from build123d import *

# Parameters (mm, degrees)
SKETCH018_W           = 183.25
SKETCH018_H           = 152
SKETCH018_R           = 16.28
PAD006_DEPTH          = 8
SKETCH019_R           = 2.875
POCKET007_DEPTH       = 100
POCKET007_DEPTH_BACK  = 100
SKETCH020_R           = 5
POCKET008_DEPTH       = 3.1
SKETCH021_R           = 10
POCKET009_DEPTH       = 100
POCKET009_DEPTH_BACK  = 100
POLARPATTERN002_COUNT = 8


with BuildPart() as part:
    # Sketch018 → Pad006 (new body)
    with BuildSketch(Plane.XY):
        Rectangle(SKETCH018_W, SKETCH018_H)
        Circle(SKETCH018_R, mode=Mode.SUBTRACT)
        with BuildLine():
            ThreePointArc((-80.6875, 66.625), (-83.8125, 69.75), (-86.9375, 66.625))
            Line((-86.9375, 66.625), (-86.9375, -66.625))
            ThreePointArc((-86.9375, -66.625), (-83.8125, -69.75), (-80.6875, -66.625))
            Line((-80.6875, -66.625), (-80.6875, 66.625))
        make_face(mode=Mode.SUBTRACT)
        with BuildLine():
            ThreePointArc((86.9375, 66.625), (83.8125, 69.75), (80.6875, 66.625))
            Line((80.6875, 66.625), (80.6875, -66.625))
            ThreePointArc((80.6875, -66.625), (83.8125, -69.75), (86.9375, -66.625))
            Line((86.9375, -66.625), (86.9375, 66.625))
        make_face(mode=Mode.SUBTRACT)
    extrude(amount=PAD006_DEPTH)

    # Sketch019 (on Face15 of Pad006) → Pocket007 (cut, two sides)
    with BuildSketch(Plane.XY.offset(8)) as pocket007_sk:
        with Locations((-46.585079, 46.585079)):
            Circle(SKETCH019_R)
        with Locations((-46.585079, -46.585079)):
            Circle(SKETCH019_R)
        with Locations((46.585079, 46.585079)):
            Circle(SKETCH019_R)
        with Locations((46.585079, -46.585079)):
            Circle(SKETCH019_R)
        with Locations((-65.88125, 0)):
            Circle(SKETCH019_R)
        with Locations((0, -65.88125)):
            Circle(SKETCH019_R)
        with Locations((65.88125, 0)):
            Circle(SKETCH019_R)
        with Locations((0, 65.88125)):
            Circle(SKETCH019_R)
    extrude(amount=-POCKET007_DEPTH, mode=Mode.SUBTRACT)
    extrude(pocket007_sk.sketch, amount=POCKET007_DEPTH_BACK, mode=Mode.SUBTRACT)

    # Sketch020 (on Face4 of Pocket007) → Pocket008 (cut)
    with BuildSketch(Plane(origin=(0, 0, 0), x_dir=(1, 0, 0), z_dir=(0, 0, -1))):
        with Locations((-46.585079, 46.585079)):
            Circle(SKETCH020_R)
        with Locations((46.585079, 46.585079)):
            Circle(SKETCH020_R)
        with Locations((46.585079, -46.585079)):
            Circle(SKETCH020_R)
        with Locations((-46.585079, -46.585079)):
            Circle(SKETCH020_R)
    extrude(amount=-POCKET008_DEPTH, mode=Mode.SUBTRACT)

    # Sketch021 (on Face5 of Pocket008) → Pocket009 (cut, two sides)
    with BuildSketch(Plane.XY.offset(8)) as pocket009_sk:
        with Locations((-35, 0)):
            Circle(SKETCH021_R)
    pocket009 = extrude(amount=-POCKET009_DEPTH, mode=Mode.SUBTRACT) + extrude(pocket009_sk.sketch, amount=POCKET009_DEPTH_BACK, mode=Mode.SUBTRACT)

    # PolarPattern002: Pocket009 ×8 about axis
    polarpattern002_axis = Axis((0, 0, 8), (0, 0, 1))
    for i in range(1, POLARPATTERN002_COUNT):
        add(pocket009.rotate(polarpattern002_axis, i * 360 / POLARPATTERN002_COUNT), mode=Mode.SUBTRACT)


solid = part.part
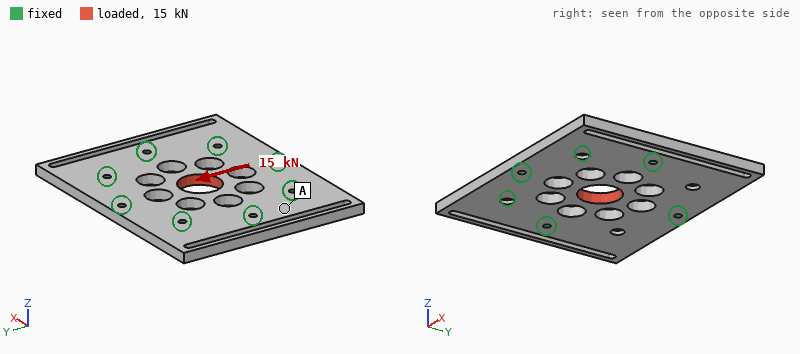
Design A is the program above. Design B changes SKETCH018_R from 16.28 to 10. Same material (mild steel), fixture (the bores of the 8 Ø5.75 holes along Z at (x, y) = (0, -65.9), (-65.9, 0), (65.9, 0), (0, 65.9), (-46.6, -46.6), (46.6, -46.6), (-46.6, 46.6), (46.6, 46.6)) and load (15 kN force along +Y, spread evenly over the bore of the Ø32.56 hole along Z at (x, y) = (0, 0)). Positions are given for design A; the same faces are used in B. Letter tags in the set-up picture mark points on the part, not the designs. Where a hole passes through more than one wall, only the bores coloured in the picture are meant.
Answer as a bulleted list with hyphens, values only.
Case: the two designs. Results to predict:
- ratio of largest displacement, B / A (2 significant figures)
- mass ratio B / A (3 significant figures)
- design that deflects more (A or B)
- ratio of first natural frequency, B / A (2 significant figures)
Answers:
- 1.1
- 1.02
- B
- 1.00
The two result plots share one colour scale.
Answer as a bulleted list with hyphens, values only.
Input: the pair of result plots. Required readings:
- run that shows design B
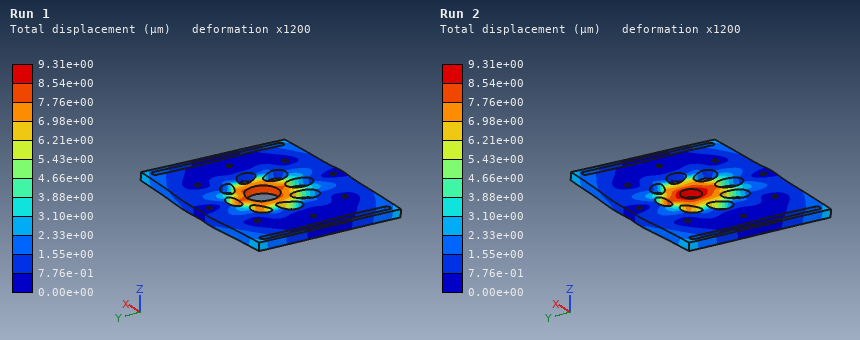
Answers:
- Run 2
